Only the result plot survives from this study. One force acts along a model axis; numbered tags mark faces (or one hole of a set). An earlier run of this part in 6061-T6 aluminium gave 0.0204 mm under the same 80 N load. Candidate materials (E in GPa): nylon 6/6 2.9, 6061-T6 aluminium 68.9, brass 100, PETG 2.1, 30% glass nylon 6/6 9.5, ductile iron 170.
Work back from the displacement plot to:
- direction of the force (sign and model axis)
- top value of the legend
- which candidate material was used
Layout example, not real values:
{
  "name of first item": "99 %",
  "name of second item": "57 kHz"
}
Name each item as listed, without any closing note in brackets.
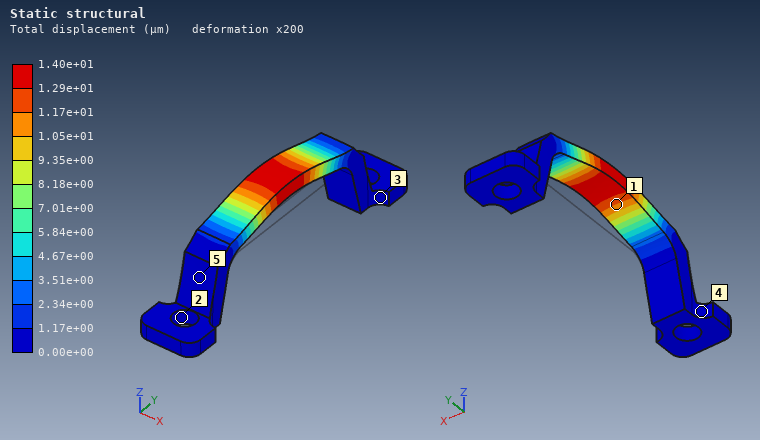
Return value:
{
  "direction of the force": "+Z",
  "top value of the legend": "1.40e+01 µm",
  "which candidate material was used": "brass"
}
